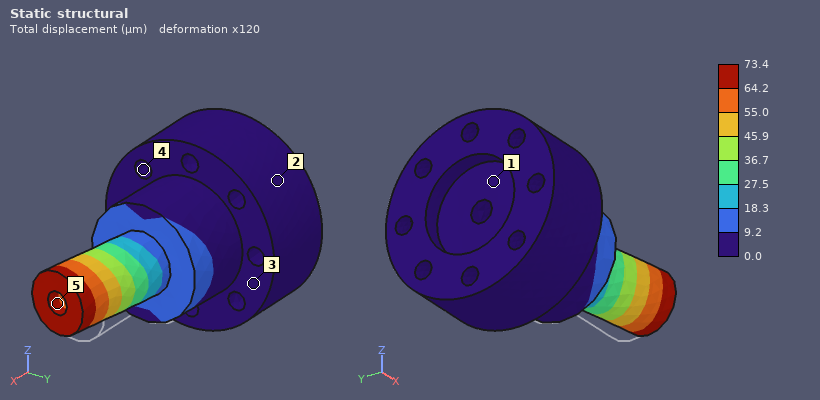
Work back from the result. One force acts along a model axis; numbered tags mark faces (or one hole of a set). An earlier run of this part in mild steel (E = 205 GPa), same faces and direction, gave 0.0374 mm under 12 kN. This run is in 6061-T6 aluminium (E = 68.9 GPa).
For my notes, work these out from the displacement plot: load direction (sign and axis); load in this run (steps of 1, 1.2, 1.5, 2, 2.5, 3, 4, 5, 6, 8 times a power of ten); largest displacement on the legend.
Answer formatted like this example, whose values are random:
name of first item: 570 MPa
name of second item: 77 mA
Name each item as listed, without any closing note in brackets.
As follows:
load direction: -Y
load in this run: 8 kN
largest displacement on the legend: 73.4 µm
